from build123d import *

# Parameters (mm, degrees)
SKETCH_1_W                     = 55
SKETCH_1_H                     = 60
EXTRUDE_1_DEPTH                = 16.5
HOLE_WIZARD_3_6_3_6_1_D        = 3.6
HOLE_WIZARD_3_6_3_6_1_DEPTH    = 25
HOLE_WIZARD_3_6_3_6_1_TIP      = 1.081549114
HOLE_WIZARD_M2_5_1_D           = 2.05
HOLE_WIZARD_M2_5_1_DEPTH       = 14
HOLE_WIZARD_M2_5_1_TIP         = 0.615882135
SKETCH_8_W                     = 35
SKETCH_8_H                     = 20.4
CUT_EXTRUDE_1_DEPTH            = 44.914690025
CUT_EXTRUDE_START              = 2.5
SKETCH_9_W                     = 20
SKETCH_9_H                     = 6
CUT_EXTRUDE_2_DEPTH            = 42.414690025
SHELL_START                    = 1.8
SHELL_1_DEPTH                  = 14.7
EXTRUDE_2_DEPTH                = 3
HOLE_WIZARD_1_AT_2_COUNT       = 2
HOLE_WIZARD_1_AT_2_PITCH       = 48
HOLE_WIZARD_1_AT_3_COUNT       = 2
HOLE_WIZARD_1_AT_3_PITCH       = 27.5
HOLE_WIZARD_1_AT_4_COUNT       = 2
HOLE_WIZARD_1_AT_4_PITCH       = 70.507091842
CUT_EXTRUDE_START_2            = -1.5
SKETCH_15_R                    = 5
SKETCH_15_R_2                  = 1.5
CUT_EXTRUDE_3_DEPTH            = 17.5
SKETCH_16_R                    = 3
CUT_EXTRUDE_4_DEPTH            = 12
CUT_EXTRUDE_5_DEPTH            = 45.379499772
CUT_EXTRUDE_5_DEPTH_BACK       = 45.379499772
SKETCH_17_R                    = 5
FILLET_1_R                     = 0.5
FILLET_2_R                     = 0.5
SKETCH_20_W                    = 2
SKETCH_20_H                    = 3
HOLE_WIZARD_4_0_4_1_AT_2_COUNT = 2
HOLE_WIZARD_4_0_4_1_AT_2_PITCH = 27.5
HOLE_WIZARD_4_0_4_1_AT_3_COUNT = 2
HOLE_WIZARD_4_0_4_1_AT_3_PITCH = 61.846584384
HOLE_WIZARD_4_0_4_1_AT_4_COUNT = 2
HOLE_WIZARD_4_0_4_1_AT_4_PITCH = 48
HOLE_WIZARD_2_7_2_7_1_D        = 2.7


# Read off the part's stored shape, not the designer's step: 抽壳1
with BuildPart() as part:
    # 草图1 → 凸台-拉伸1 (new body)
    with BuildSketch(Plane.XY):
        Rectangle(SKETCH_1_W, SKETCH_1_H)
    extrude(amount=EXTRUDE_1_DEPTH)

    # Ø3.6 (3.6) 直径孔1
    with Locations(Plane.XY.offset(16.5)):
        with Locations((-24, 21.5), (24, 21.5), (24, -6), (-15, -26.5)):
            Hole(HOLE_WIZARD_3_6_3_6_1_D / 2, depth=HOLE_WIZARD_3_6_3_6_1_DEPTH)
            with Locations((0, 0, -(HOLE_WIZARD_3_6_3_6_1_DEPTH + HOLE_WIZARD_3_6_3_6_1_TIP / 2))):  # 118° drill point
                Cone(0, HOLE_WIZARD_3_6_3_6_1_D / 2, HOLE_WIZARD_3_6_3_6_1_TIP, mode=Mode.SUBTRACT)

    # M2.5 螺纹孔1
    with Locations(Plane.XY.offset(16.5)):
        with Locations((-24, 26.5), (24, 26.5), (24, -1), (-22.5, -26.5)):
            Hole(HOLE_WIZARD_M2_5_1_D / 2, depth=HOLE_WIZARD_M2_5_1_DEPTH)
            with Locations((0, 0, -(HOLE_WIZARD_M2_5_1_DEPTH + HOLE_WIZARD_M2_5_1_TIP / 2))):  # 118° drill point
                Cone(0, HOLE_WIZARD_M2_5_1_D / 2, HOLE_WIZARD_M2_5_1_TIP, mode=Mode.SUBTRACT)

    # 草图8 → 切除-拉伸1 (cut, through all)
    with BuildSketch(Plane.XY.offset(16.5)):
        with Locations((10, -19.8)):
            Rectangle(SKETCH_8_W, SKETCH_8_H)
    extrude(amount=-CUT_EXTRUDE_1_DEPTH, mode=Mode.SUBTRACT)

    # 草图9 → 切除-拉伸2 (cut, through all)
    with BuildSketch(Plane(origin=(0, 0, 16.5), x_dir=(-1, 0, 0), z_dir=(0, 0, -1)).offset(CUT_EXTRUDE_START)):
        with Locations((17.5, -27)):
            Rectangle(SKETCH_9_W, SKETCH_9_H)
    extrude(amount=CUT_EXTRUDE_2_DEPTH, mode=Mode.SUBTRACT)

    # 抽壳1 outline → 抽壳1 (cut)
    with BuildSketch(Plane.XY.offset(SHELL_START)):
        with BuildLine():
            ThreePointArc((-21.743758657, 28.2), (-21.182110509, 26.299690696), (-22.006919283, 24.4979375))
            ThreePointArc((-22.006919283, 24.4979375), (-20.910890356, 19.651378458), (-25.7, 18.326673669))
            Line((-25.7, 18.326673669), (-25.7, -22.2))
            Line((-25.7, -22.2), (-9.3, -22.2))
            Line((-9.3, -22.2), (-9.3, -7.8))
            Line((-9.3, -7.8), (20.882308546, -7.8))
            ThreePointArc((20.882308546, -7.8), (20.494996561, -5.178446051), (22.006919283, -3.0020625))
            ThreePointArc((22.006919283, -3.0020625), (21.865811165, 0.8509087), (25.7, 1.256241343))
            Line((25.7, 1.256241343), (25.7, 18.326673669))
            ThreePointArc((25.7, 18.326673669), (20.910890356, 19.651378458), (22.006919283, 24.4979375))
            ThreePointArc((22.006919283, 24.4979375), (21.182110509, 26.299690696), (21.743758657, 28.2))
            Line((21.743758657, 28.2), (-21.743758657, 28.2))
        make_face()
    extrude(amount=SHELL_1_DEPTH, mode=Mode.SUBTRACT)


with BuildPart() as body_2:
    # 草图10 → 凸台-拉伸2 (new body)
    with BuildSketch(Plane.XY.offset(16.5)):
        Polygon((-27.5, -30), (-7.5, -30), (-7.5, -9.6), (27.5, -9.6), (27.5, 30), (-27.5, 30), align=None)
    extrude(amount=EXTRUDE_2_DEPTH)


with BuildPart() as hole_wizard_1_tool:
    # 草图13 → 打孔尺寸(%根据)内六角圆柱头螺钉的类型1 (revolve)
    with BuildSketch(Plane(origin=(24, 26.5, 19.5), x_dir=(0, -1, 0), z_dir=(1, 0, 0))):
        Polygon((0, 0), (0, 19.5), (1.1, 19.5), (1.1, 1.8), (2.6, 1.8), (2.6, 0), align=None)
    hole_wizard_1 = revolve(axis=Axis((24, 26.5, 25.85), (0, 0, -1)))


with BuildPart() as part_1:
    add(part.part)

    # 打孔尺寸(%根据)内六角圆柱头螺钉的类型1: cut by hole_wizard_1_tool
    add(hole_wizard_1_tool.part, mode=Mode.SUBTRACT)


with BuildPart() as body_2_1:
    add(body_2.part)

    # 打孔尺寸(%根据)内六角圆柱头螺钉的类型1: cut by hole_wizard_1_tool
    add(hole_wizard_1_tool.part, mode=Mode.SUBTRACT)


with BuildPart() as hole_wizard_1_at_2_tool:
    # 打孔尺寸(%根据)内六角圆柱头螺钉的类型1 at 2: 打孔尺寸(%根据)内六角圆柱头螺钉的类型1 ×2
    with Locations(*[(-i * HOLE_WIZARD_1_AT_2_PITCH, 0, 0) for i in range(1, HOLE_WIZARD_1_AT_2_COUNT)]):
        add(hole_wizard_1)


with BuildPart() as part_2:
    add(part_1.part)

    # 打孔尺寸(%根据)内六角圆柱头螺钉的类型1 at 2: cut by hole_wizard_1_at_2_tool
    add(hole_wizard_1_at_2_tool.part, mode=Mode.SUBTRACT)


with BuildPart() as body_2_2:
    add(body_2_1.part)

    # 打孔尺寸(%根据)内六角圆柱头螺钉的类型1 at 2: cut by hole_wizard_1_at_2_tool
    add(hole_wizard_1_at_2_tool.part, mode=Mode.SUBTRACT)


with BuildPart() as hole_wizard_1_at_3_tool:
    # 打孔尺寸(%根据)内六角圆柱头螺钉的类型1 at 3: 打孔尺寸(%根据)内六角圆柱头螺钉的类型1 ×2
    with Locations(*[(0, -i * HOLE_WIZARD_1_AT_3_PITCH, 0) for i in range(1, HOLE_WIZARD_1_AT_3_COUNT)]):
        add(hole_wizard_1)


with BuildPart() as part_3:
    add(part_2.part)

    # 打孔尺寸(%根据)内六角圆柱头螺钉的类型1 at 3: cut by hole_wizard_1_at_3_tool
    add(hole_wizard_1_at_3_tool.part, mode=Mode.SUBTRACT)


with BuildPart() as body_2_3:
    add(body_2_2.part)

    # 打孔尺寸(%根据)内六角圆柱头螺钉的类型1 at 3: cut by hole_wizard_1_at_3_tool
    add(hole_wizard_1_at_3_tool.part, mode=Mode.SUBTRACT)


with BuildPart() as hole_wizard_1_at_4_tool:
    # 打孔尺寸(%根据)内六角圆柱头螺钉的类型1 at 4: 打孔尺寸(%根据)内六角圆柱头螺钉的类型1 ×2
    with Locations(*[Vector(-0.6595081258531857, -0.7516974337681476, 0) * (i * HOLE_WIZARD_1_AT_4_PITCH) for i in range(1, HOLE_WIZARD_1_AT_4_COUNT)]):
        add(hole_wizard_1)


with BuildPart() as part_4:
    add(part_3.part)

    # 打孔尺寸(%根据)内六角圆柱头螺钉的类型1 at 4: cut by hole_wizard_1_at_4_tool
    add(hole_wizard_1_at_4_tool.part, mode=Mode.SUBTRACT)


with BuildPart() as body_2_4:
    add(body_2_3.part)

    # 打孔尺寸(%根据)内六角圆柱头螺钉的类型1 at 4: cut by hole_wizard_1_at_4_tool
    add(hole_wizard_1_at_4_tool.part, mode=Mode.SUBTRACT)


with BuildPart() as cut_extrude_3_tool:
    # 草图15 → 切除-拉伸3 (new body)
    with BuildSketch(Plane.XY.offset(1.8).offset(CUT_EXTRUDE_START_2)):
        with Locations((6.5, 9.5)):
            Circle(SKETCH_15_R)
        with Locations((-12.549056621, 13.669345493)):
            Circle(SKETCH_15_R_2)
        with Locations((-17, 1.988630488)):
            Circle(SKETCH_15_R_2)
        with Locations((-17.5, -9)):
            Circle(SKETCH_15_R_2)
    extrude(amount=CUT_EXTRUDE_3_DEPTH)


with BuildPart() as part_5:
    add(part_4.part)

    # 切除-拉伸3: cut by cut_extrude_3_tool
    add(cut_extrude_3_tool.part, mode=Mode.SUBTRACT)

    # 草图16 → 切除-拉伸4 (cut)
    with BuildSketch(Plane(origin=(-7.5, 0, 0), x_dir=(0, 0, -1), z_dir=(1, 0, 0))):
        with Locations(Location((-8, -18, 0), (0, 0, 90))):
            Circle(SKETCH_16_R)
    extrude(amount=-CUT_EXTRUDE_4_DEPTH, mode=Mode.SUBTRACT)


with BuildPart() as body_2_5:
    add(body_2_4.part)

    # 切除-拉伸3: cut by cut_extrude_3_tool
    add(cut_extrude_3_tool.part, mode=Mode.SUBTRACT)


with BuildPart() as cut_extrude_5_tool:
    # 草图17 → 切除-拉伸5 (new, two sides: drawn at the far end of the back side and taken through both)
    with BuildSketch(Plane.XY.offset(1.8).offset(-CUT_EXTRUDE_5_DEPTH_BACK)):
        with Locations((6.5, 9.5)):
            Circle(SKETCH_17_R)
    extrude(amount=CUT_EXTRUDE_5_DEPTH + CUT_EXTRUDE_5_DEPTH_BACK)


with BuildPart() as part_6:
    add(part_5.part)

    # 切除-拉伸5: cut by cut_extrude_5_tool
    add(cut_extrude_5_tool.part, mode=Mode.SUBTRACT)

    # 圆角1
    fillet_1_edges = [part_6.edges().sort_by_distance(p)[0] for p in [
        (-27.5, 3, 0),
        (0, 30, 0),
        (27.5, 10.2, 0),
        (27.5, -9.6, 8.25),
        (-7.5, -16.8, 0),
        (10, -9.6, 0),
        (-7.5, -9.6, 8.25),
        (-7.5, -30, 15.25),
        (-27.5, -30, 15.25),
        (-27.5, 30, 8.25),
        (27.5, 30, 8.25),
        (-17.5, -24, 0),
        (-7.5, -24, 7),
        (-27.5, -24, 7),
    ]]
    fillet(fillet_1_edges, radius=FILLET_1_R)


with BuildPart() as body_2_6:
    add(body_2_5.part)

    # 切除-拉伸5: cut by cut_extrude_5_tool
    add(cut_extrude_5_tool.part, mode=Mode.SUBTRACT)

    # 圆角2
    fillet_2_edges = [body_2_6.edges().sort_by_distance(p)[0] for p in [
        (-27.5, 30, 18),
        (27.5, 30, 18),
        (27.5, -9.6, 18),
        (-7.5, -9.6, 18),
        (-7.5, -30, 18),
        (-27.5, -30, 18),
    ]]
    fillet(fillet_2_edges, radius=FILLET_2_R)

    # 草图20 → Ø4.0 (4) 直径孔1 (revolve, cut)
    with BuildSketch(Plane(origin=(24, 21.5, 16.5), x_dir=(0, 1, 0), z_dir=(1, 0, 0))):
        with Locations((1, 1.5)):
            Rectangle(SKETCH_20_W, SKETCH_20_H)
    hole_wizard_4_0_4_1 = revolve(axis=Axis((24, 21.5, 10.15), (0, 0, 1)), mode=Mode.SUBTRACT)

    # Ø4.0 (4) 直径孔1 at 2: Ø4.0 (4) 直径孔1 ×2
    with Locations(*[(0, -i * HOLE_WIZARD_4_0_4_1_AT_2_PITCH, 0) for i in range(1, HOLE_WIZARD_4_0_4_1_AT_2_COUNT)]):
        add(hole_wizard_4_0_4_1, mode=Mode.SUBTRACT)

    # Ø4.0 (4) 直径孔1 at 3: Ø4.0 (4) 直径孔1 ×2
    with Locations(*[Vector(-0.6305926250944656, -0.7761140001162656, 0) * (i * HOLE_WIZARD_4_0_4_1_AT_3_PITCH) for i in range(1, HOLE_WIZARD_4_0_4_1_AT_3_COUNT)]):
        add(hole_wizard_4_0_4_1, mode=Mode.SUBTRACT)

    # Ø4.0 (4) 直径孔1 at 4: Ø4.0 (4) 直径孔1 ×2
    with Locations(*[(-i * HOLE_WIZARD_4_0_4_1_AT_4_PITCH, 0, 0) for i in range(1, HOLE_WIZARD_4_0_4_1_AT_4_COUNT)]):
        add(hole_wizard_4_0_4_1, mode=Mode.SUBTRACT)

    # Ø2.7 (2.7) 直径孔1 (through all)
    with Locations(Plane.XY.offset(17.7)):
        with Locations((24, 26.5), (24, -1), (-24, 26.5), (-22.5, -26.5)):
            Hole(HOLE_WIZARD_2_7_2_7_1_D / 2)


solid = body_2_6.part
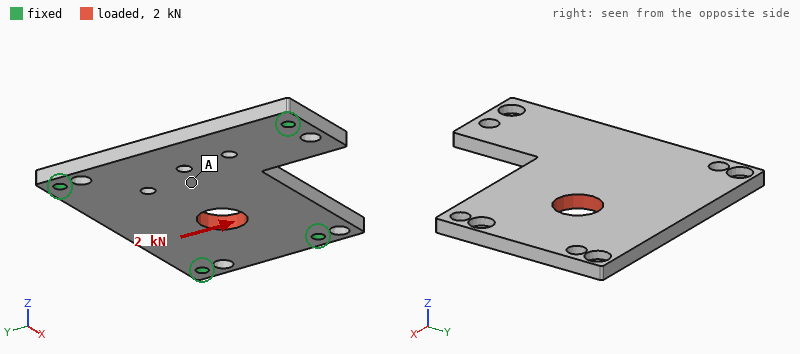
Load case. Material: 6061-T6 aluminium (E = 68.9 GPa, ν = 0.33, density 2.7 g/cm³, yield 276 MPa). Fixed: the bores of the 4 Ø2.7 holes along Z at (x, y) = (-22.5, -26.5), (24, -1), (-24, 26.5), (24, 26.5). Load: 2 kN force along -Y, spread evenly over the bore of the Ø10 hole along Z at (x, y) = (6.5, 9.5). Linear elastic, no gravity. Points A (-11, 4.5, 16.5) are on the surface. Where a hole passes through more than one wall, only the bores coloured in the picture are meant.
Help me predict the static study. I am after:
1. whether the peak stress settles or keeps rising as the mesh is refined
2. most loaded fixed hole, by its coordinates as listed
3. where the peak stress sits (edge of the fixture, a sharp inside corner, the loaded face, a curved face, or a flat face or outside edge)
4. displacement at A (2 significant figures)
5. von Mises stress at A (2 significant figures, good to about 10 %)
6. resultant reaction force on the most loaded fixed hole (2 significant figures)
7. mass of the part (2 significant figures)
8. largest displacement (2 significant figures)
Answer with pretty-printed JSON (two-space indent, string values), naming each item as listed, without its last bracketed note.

{
  "whether the peak stress settles or keeps rising as the mesh is refined": "keeps rising",
  "most loaded fixed hole, by its coordinates as listed": "(24, -1)",
  "where the peak stress sits": "edge of the fixture",
  "displacement at A": "8.3 µm",
  "von Mises stress at A": "12 MPa",
  "resultant reaction force on the most loaded fixed hole": "720 N",
  "mass of the part": "19 g",
  "largest displacement": "14 µm"
}
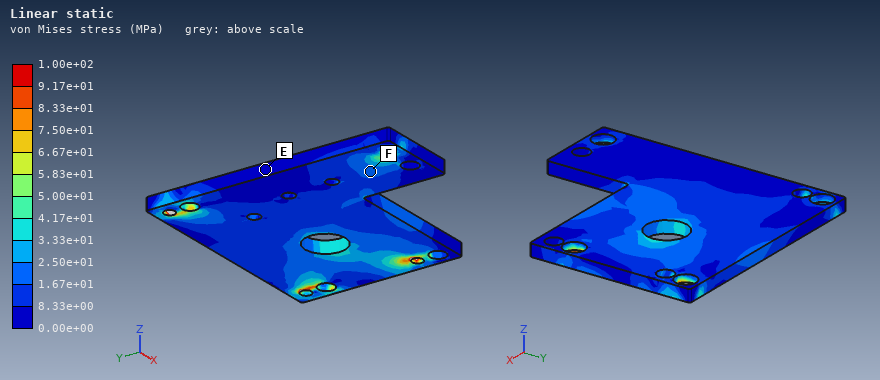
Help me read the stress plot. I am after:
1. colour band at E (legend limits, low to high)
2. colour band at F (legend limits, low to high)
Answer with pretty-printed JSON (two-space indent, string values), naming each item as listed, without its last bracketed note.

{
  "colour band at E": "0.00e+00 to 8.33e+00 MPa",
  "colour band at F": "1.67e+01 to 2.50e+01 MPa"
}
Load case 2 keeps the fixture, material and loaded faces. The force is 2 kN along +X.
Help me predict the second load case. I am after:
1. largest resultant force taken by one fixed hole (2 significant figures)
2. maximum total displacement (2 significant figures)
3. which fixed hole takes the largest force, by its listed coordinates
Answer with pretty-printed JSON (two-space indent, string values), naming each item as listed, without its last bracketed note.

{
  "largest resultant force taken by one fixed hole": "810 N",
  "maximum total displacement": "15 µm",
  "which fixed hole takes the largest force, by its listed coordinates": "(24, -1)"
}
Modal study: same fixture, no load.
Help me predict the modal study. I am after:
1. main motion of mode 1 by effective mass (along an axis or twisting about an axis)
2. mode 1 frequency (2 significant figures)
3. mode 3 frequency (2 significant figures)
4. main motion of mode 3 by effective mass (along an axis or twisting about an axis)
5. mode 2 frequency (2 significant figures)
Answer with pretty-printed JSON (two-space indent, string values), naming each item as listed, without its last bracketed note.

{
  "main motion of mode 1 by effective mass": "along Z",
  "mode 1 frequency": "3500 Hz",
  "mode 3 frequency": "6600 Hz",
  "main motion of mode 3 by effective mass": "twisting about X",
  "mode 2 frequency": "5600 Hz"
}
